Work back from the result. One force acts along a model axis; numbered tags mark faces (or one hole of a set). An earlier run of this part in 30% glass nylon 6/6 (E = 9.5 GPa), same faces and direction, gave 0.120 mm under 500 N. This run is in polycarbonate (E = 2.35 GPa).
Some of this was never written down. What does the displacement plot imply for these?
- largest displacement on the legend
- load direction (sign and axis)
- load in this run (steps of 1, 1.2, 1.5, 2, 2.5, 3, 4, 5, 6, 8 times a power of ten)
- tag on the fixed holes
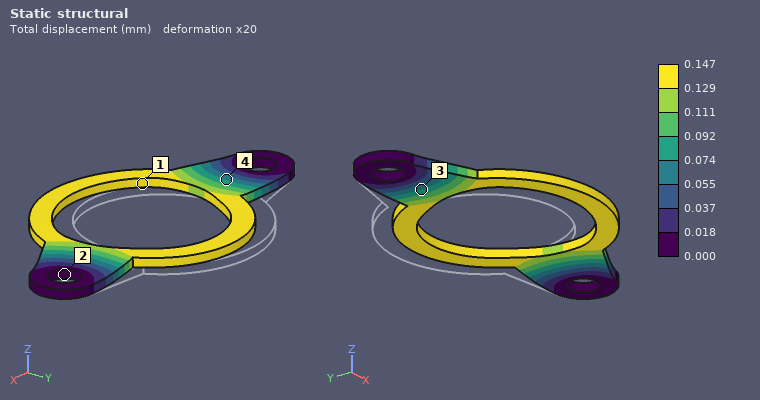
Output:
0.147 mm
-Y
150 N
2
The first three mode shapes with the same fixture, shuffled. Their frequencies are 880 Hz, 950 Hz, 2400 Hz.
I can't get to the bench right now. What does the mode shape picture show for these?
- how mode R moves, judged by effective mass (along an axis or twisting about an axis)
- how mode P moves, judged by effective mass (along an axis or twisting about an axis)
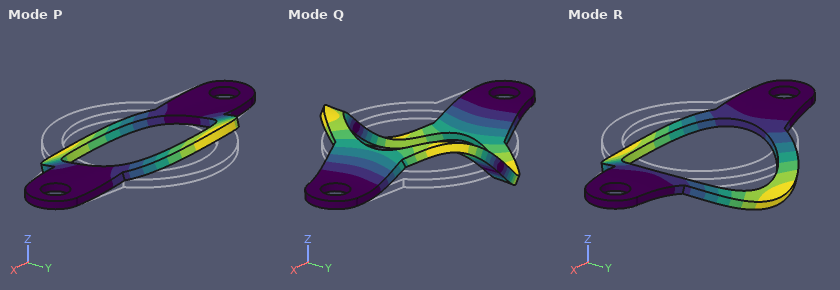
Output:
along Z
twisting about X
